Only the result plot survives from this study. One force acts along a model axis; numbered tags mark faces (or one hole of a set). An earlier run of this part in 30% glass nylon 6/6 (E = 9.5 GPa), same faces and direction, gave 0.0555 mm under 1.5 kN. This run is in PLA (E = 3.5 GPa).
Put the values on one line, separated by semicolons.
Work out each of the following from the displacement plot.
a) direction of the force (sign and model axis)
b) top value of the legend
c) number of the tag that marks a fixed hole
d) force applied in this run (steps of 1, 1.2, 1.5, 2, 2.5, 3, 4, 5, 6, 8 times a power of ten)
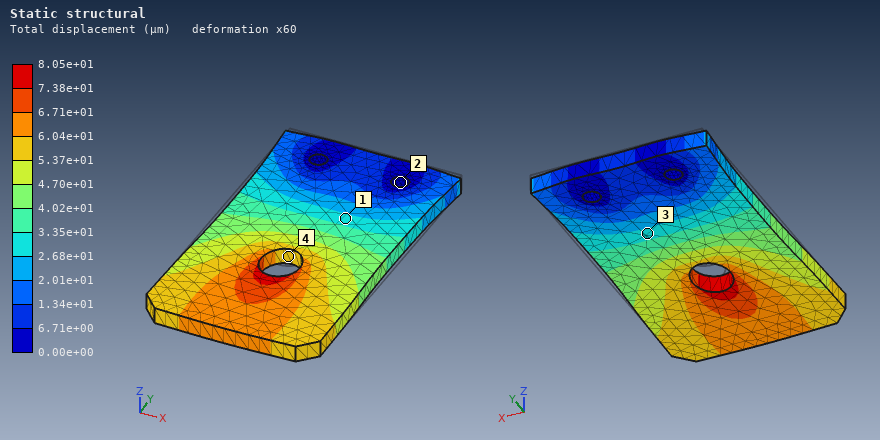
-Y; 8.05e+01 µm; 2; 800 N
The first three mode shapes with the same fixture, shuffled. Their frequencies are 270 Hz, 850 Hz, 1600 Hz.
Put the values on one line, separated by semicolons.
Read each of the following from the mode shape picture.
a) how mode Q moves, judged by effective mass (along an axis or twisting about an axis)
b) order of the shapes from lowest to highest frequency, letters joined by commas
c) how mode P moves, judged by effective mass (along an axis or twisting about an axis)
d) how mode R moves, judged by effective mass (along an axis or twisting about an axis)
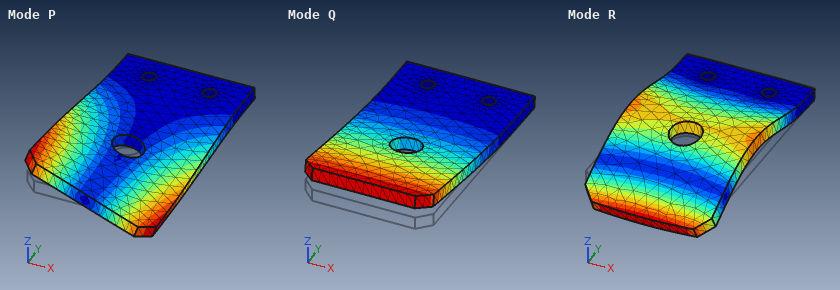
along Z; Q, P, R; twisting about Y; along Z
